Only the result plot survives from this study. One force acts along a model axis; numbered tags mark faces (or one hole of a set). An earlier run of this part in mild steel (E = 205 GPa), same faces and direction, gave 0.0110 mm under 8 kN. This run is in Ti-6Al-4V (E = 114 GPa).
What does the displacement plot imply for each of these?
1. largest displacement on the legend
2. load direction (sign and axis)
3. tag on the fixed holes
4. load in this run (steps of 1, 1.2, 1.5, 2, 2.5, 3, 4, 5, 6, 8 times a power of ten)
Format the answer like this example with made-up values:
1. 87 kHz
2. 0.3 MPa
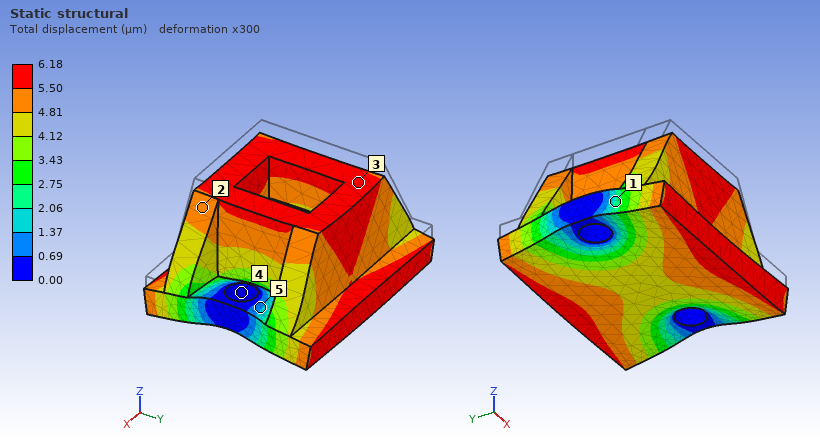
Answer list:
1. 6.18 µm
2. -Z
3. 4
4. 2.5 kN
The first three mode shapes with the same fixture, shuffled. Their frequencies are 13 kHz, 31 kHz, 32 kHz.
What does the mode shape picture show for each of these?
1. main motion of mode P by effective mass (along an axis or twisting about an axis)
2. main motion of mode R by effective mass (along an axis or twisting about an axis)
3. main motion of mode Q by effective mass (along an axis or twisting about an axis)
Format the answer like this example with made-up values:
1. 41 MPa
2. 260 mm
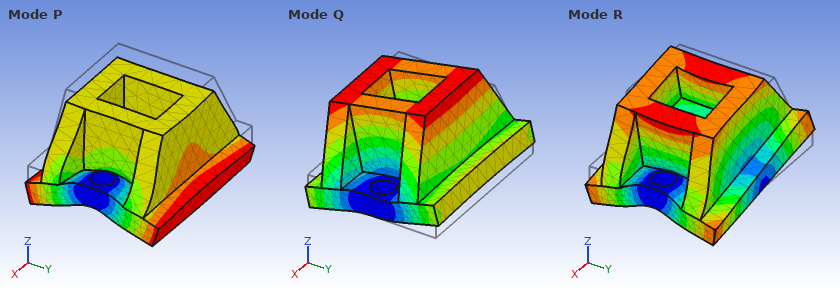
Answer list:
1. along Z
2. along X
3. along Y
